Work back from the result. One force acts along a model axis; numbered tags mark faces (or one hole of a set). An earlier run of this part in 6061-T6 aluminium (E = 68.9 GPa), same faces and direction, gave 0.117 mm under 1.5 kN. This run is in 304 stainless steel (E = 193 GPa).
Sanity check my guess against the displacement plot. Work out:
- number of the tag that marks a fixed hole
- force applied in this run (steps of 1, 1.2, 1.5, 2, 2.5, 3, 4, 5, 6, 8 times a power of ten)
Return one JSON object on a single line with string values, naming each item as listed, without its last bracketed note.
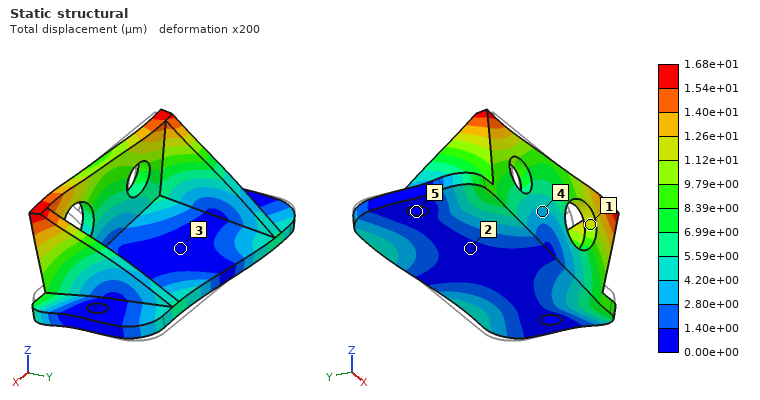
{"number of the tag that marks a fixed hole": "5", "force applied in this run": "600 N"}
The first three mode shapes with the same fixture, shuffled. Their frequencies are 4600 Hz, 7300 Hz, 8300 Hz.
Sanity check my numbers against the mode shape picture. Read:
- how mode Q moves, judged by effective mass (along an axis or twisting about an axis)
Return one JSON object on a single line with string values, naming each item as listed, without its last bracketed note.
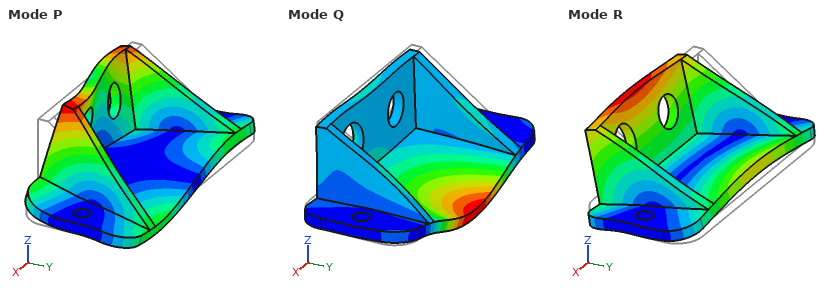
{"how mode Q moves, judged by effective mass": "along Z"}
